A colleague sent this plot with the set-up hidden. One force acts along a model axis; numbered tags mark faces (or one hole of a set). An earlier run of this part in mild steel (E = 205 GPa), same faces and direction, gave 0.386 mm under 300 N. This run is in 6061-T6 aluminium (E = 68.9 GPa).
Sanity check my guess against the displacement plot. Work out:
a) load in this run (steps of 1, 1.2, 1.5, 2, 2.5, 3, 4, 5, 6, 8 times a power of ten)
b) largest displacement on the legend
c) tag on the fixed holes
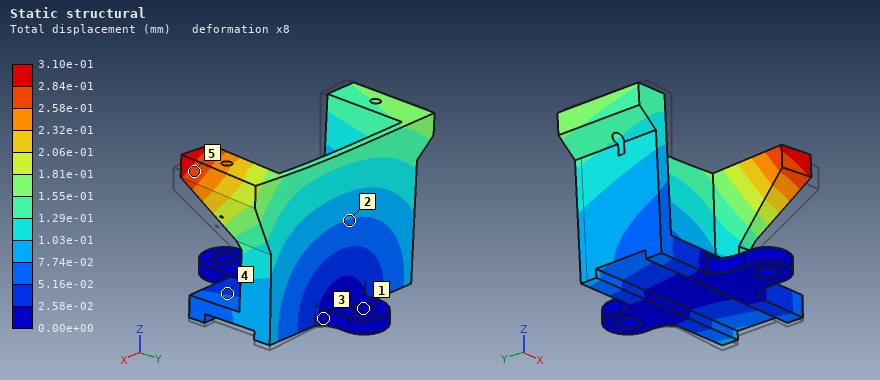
80 N
3.10e-01 mm
1
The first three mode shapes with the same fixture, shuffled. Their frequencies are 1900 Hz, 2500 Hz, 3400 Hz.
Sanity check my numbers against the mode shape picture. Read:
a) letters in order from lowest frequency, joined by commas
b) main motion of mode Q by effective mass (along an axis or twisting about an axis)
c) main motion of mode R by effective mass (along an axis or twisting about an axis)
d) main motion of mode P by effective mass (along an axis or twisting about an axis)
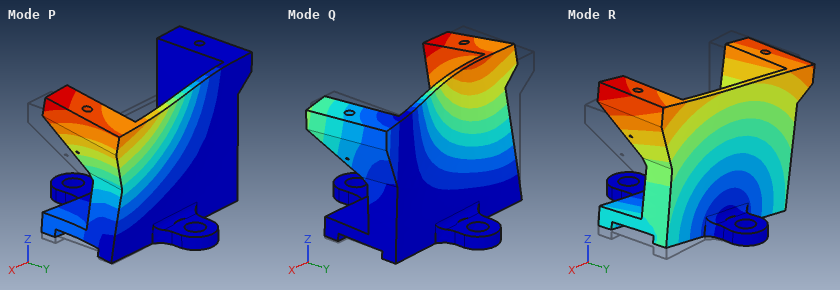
R, P, Q
along Y
along X
along Y
